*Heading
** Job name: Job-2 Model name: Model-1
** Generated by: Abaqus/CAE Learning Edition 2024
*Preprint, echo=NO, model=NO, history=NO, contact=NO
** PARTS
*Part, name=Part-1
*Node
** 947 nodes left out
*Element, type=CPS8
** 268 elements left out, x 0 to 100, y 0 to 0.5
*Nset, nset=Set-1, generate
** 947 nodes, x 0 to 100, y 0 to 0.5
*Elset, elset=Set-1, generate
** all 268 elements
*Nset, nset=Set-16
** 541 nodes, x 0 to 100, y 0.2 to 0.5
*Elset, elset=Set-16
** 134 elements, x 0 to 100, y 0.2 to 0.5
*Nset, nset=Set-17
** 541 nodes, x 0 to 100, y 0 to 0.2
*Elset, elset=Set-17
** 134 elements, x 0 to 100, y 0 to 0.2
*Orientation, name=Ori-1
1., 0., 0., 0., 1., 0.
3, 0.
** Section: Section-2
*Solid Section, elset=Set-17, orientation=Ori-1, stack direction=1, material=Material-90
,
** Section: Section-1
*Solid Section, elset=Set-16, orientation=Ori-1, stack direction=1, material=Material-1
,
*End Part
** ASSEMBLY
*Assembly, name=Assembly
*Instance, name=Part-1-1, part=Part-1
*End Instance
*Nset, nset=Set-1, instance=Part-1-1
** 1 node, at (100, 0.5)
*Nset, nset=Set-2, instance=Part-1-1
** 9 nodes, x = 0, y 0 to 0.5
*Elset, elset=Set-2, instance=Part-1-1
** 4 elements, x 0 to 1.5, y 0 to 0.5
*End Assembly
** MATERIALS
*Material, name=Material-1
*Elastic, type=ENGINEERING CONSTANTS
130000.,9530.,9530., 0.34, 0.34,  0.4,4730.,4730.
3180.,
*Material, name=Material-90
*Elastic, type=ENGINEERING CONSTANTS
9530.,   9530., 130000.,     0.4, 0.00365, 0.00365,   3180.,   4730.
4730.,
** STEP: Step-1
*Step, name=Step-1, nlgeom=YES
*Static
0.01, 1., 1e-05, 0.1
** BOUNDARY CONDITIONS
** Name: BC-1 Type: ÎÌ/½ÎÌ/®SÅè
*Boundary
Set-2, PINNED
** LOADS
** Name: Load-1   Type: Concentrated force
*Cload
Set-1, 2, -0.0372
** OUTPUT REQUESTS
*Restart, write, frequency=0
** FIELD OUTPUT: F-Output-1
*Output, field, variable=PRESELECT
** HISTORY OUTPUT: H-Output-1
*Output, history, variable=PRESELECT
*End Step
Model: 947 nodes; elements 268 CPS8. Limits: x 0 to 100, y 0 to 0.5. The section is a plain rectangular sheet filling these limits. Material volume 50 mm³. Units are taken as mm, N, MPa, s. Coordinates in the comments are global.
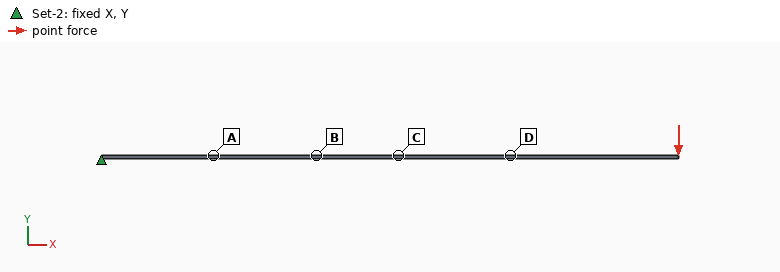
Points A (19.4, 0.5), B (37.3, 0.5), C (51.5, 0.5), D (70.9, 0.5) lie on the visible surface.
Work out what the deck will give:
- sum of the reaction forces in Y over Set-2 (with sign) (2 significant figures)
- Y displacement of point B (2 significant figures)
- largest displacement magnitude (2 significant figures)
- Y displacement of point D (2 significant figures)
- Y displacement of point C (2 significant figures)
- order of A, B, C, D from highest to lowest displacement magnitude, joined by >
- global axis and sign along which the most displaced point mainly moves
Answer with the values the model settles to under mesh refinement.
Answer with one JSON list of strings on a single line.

["0.037 N", "-6.4 mm", "35 mm", "-20 mm", "-11 mm", "D > C > B > A", "-Y"]
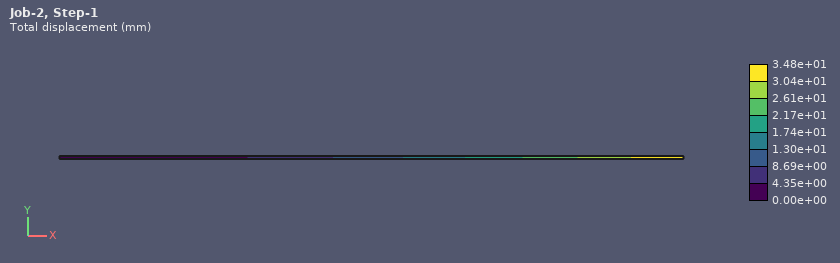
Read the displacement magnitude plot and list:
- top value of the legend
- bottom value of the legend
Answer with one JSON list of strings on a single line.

["3.48e+01 mm", "0.00e+00 mm"]
